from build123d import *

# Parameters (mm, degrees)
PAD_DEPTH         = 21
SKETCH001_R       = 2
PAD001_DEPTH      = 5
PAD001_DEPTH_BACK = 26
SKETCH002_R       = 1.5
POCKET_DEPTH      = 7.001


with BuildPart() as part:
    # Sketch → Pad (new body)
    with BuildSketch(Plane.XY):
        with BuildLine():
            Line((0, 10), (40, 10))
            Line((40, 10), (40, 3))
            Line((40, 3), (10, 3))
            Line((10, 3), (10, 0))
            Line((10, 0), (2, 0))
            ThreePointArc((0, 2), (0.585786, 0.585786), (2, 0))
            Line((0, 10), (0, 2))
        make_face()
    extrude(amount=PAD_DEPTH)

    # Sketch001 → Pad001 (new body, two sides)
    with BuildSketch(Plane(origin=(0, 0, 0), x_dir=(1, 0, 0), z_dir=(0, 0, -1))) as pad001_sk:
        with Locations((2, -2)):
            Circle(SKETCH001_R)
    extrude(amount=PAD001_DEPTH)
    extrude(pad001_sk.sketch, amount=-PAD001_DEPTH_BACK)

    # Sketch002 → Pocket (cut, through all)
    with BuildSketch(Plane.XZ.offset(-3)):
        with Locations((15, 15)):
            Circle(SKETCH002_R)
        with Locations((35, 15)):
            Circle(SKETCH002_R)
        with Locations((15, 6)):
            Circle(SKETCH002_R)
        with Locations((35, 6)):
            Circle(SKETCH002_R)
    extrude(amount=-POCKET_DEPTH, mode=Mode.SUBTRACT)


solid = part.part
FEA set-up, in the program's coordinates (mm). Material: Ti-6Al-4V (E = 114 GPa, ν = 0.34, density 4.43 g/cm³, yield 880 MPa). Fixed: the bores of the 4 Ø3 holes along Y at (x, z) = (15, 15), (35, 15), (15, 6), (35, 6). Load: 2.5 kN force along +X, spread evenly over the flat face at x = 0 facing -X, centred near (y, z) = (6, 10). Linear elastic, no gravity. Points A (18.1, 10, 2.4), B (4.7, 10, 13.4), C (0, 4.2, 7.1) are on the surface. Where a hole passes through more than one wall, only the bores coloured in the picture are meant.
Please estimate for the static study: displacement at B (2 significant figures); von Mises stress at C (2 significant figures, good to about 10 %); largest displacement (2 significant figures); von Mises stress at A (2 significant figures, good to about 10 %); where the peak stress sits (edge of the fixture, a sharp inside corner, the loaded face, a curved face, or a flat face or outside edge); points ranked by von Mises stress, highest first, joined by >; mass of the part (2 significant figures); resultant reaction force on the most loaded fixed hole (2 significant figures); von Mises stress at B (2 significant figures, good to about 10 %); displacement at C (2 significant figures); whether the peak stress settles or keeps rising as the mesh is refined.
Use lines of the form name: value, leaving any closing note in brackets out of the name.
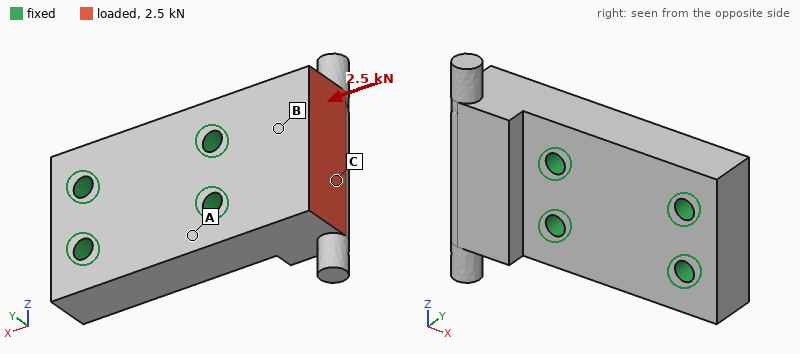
displacement at B: 1.4 µm
von Mises stress at C: 12 MPa
largest displacement: 2.8 µm
von Mises stress at A: 4.8 MPa
where the peak stress sits: edge of the fixture
points ranked by von Mises stress, highest first, joined by >: B > C > A
mass of the part: 28 g
resultant reaction force on the most loaded fixed hole: 1.2 kN
von Mises stress at B: 17 MPa
displacement at C: 2.5 µm
whether the peak stress settles or keeps rising as the mesh is refined: keeps rising
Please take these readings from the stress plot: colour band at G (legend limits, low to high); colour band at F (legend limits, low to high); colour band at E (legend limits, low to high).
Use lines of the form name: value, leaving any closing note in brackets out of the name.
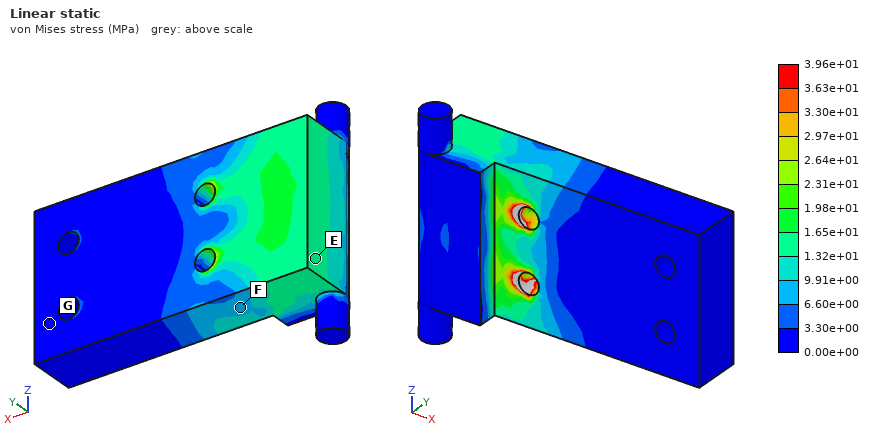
colour band at G: 0.00e+00 to 3.30e+00 MPa
colour band at F: 6.60e+00 to 9.91e+00 MPa
colour band at E: 1.32e+01 to 1.65e+01 MPa
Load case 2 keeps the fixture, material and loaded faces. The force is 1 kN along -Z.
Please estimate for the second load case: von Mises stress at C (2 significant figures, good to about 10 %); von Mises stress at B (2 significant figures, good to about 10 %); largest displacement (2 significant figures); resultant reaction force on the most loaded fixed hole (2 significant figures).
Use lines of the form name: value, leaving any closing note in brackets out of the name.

von Mises stress at C: 11 MPa
von Mises stress at B: 19 MPa
largest displacement: 7.1 µm
resultant reaction force on the most loaded fixed hole: 1.1 kN
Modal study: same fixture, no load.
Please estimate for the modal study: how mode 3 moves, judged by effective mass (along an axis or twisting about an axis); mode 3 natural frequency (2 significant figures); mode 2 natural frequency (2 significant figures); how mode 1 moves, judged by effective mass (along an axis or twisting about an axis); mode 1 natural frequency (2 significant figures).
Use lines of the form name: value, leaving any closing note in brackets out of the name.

how mode 3 moves, judged by effective mass: along Z
mode 3 natural frequency: 29 kHz
mode 2 natural frequency: 26 kHz
how mode 1 moves, judged by effective mass: along Y
mode 1 natural frequency: 18 kHz
